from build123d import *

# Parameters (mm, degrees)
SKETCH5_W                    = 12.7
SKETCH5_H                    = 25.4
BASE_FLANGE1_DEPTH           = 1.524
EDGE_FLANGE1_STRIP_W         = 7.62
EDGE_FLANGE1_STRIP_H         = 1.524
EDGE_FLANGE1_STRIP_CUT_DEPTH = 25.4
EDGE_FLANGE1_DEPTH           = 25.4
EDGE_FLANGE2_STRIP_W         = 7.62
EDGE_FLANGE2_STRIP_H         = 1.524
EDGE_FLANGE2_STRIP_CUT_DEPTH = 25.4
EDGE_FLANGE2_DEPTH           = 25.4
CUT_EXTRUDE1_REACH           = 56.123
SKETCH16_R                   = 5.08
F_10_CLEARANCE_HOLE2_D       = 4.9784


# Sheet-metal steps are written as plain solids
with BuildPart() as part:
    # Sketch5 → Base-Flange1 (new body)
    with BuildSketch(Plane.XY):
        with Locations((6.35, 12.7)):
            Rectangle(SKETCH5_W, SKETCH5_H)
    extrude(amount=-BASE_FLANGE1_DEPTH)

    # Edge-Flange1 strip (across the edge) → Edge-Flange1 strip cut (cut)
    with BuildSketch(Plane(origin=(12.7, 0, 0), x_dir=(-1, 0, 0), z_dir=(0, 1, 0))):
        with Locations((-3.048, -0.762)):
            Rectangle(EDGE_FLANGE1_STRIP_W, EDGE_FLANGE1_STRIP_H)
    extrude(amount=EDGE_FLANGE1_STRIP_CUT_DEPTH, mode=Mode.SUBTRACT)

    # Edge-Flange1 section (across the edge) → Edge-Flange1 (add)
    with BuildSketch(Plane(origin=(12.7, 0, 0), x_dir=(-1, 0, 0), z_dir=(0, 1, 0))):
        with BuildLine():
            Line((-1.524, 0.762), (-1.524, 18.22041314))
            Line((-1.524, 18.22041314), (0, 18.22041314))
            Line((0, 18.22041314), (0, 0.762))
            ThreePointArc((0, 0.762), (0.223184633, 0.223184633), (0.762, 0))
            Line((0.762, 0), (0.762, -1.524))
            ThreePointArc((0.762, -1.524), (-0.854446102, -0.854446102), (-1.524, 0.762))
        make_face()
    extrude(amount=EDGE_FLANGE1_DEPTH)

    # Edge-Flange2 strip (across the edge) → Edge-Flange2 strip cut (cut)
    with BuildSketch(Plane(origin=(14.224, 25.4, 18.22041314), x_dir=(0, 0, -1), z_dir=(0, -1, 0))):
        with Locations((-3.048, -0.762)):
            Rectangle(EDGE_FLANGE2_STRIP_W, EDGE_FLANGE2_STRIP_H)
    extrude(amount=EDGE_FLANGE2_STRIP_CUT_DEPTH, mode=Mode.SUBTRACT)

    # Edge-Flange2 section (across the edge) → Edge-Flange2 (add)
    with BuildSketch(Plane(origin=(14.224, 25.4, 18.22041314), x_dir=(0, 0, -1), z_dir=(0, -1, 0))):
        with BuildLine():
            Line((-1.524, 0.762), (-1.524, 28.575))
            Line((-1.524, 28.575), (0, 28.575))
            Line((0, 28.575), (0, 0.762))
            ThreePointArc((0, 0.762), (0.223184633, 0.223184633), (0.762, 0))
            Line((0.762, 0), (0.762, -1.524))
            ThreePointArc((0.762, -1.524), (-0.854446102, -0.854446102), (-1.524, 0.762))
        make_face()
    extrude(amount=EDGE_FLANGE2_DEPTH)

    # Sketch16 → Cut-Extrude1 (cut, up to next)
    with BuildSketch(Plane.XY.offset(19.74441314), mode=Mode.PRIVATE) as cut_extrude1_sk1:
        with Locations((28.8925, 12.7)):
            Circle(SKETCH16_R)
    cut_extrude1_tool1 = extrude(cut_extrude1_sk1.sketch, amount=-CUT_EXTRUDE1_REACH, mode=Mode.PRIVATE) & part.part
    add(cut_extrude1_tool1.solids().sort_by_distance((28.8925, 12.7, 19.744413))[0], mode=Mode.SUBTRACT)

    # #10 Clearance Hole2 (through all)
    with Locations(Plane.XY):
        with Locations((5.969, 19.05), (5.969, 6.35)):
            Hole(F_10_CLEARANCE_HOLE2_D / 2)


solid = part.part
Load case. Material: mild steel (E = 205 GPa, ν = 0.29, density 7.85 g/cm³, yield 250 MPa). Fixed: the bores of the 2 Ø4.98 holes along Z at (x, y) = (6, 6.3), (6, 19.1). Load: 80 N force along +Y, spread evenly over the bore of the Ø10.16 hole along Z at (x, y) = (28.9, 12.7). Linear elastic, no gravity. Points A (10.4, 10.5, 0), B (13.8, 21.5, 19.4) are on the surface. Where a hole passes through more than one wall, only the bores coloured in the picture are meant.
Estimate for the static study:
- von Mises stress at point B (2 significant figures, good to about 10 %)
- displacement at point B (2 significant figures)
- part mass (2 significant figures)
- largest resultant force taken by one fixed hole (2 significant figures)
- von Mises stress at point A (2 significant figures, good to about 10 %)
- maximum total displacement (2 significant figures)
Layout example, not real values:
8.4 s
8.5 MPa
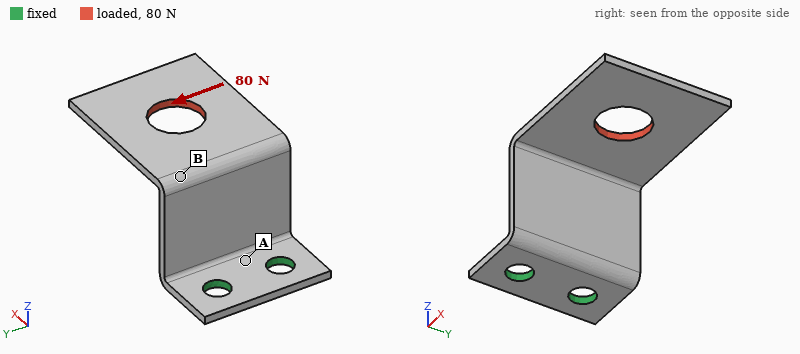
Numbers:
55 MPa
0.056 mm
17 g
150 N
15 MPa
0.21 mm
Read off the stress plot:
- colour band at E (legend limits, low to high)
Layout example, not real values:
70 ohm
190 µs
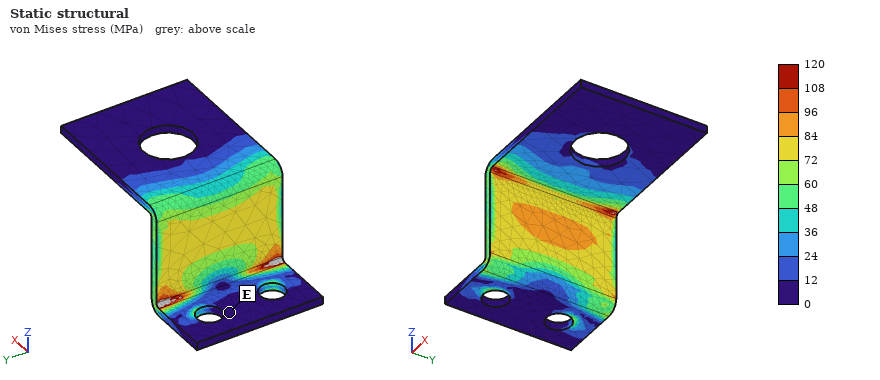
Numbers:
0 to 12 MPa
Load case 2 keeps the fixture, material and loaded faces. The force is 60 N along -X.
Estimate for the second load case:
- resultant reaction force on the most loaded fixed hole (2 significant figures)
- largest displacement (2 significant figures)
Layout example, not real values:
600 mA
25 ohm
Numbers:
32 N
0.38 mm
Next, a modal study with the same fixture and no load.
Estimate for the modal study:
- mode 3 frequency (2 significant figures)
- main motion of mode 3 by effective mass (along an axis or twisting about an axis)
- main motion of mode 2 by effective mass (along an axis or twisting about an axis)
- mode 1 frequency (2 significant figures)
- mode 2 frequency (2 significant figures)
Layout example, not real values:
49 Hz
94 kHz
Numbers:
1800 Hz
along X
along Y
610 Hz
1300 Hz
